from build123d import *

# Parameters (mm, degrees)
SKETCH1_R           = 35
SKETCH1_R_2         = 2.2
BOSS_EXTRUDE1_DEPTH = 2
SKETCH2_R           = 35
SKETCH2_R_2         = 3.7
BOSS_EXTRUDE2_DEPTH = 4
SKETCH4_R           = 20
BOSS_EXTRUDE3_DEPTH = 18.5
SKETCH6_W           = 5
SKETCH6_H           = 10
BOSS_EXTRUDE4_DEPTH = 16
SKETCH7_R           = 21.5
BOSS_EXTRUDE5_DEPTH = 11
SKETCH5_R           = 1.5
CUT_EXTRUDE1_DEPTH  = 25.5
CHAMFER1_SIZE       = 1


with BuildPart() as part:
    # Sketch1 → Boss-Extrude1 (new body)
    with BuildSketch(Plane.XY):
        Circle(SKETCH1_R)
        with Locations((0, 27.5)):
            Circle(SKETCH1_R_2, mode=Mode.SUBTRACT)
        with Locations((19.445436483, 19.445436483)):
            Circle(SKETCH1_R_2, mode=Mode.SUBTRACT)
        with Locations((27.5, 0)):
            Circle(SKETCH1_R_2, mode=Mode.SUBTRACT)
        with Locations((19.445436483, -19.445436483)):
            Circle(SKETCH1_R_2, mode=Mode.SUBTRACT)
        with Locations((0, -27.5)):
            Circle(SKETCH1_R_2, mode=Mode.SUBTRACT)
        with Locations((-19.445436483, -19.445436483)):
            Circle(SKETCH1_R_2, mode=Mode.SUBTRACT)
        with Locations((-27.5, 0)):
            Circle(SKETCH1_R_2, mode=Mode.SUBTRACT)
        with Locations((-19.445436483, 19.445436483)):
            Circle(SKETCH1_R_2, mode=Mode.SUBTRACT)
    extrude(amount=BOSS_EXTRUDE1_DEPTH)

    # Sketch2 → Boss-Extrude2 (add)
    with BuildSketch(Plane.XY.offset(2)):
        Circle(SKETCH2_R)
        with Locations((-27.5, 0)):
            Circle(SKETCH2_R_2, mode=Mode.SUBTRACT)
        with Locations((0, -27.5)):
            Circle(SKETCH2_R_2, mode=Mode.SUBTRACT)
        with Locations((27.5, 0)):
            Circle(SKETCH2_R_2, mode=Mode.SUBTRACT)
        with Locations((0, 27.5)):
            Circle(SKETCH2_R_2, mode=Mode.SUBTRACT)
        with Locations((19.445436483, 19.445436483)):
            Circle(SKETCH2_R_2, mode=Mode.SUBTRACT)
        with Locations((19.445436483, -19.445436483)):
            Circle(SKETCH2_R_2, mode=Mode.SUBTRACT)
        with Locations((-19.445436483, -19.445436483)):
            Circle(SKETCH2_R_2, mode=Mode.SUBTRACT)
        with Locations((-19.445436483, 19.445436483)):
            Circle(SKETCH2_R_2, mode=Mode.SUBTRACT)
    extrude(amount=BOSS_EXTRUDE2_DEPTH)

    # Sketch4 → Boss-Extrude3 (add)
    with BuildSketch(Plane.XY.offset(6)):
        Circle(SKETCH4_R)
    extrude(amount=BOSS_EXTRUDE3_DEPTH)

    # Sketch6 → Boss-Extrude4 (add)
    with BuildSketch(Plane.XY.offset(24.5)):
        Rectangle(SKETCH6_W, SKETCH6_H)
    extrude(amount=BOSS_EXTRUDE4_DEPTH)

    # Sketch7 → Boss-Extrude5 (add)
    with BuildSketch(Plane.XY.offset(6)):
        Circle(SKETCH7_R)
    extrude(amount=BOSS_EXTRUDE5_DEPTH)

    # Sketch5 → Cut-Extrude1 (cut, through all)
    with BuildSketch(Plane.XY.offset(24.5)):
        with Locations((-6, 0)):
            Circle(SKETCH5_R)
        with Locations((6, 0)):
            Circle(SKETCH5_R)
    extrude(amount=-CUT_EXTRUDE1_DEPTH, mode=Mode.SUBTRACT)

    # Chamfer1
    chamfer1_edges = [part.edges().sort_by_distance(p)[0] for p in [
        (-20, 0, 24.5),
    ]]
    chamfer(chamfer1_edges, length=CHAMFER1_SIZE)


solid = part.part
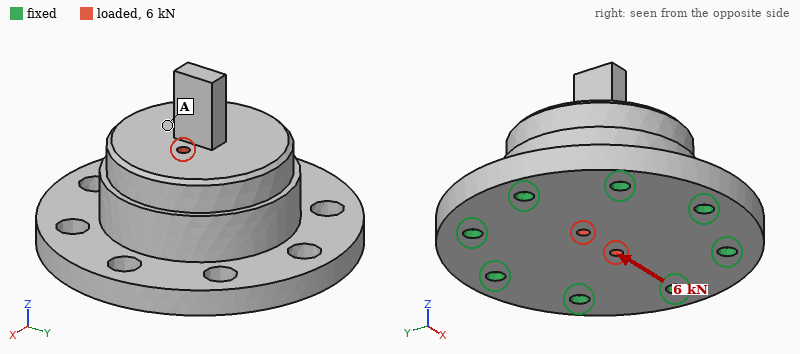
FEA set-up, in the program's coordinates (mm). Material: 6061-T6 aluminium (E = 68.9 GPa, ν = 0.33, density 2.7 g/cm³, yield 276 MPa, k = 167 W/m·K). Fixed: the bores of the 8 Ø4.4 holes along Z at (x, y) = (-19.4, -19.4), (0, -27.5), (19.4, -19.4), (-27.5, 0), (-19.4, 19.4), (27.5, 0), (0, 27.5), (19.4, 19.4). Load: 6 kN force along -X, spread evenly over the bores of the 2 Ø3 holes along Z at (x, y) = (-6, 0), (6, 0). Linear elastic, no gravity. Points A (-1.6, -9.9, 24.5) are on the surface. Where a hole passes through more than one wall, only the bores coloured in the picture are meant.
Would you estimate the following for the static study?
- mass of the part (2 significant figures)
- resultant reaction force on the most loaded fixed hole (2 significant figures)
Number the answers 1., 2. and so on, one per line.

1. 130 g
2. 1.3 kN
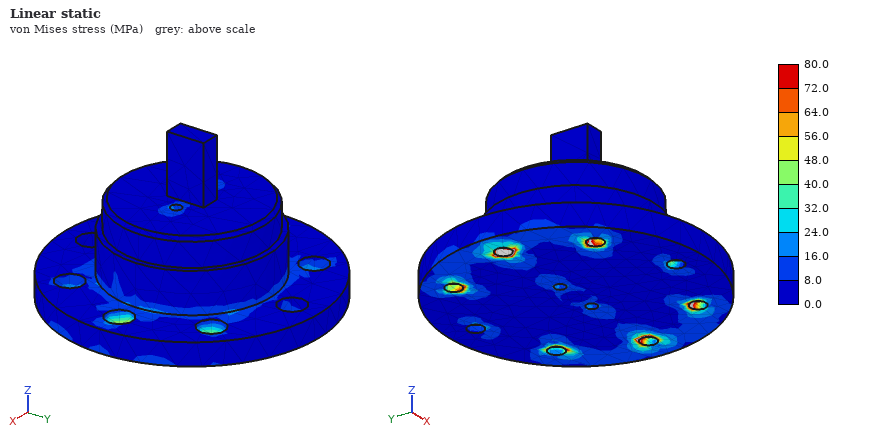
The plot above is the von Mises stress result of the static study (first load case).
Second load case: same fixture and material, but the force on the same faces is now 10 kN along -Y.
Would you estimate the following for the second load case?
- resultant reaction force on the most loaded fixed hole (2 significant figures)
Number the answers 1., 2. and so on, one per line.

1. 2.1 kN
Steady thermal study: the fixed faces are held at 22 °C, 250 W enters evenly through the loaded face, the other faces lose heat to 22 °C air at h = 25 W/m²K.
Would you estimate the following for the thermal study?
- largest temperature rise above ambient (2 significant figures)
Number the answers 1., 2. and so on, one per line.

1. 48 K
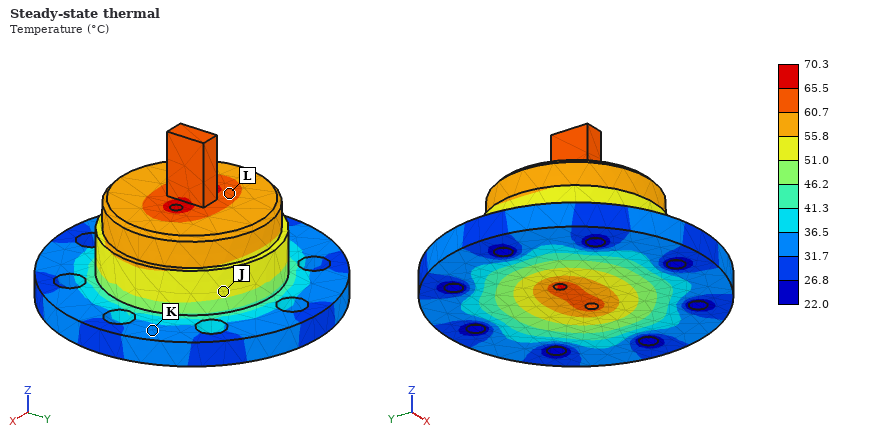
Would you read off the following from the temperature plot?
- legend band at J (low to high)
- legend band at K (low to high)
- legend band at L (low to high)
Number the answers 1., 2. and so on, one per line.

1. 51.0 to 55.8 °C
2. 31.7 to 36.5 °C
3. 60.7 to 65.5 °C
